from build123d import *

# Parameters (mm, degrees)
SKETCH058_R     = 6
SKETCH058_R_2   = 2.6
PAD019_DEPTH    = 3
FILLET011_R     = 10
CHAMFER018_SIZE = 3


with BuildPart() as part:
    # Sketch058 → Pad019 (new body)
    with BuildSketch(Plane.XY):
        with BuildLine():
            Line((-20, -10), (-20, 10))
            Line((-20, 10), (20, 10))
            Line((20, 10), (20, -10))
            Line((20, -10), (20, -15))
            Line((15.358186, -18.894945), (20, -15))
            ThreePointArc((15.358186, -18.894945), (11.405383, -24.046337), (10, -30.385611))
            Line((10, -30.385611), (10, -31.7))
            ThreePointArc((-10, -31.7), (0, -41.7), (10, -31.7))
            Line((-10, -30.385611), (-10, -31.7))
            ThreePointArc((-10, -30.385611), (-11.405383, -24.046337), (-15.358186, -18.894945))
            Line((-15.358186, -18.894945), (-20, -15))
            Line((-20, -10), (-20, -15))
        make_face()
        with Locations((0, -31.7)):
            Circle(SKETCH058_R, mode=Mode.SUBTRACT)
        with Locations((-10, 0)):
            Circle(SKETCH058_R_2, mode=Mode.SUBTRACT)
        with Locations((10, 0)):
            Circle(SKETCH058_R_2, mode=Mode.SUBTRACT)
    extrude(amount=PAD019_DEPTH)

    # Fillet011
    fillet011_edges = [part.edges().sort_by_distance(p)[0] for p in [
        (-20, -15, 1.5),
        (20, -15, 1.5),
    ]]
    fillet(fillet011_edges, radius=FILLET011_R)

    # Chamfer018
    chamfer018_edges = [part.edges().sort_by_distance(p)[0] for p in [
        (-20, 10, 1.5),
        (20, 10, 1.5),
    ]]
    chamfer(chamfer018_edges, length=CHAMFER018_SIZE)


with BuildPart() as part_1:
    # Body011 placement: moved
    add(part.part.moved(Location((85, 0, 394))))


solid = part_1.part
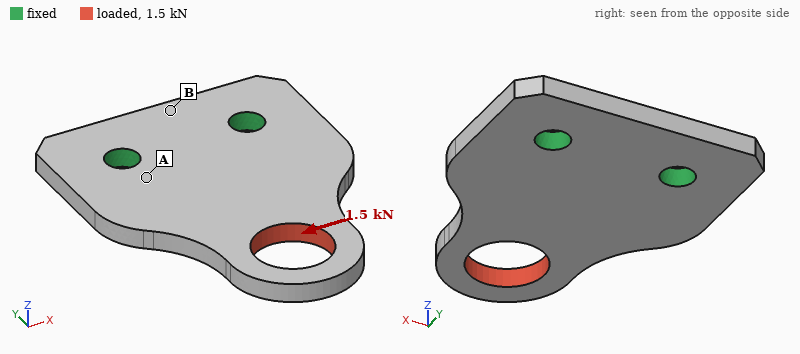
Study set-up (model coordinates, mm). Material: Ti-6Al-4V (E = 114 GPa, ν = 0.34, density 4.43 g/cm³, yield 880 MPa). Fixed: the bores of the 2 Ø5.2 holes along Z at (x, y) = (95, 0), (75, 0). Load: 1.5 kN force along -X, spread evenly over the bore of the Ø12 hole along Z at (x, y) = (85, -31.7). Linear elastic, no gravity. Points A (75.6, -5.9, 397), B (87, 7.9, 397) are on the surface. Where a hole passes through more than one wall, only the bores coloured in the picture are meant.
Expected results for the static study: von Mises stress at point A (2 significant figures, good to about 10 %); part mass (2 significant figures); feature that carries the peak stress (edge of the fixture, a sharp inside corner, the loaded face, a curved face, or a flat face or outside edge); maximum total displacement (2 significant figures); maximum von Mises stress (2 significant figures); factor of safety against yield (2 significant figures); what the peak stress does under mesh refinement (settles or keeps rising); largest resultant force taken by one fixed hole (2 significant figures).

58 MPa
19 g
the loaded face
63 µm
180 MPa
4.9
settles
2.1 kN
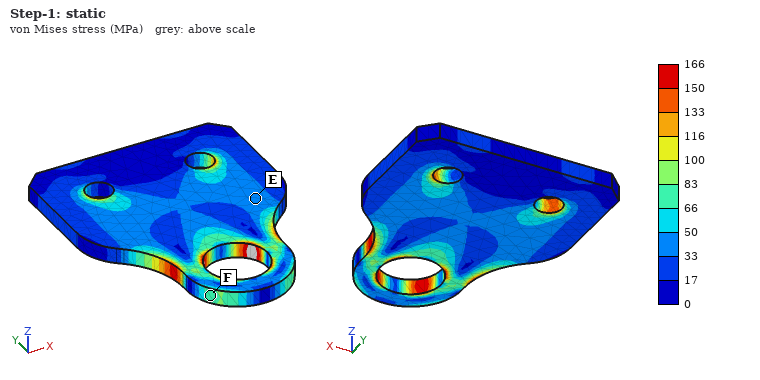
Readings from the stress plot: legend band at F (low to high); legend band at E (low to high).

66 to 83 MPa
33 to 50 MPa
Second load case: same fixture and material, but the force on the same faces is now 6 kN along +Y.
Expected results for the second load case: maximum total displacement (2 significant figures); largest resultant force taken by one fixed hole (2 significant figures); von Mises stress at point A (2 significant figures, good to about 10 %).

48 µm
3.1 kN
88 MPa
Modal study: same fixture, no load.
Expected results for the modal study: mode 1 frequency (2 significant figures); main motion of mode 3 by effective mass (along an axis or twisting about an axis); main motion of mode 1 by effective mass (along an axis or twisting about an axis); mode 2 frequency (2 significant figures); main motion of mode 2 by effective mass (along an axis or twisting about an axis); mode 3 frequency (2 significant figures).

2500 Hz
along Z
along Z
7600 Hz
twisting about Y
9100 Hz
